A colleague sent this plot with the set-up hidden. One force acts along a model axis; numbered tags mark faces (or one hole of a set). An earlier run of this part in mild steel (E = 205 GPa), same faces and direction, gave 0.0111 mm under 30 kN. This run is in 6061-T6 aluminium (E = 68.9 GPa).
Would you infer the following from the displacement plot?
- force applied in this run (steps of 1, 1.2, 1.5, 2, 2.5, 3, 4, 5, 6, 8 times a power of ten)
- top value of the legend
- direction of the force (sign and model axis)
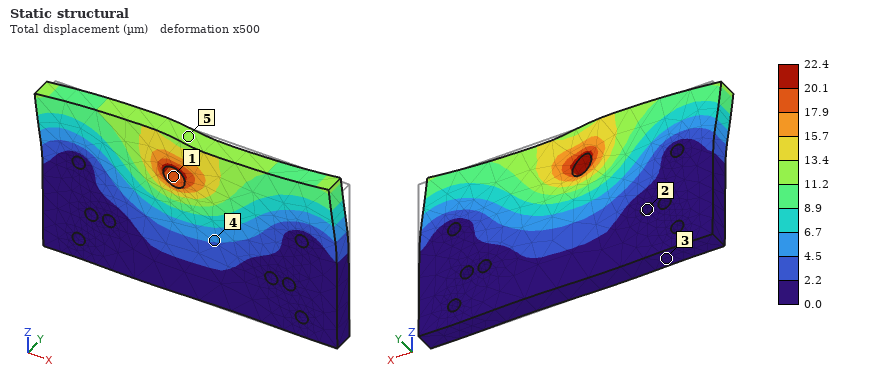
20 kN
22.4 µm
-X
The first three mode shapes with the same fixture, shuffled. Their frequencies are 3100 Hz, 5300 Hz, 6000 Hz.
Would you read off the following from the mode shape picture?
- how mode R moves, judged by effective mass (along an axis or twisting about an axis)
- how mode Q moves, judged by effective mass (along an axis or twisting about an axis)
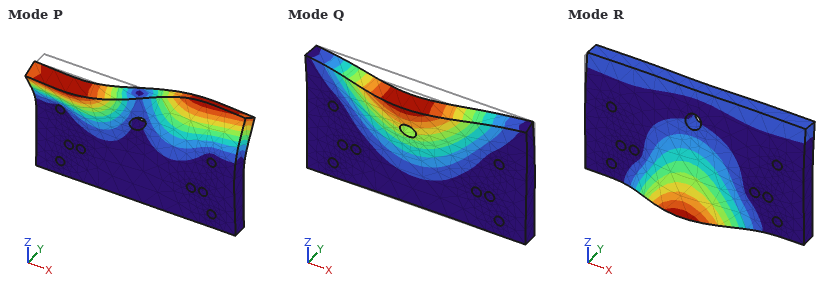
along Y
along Y
